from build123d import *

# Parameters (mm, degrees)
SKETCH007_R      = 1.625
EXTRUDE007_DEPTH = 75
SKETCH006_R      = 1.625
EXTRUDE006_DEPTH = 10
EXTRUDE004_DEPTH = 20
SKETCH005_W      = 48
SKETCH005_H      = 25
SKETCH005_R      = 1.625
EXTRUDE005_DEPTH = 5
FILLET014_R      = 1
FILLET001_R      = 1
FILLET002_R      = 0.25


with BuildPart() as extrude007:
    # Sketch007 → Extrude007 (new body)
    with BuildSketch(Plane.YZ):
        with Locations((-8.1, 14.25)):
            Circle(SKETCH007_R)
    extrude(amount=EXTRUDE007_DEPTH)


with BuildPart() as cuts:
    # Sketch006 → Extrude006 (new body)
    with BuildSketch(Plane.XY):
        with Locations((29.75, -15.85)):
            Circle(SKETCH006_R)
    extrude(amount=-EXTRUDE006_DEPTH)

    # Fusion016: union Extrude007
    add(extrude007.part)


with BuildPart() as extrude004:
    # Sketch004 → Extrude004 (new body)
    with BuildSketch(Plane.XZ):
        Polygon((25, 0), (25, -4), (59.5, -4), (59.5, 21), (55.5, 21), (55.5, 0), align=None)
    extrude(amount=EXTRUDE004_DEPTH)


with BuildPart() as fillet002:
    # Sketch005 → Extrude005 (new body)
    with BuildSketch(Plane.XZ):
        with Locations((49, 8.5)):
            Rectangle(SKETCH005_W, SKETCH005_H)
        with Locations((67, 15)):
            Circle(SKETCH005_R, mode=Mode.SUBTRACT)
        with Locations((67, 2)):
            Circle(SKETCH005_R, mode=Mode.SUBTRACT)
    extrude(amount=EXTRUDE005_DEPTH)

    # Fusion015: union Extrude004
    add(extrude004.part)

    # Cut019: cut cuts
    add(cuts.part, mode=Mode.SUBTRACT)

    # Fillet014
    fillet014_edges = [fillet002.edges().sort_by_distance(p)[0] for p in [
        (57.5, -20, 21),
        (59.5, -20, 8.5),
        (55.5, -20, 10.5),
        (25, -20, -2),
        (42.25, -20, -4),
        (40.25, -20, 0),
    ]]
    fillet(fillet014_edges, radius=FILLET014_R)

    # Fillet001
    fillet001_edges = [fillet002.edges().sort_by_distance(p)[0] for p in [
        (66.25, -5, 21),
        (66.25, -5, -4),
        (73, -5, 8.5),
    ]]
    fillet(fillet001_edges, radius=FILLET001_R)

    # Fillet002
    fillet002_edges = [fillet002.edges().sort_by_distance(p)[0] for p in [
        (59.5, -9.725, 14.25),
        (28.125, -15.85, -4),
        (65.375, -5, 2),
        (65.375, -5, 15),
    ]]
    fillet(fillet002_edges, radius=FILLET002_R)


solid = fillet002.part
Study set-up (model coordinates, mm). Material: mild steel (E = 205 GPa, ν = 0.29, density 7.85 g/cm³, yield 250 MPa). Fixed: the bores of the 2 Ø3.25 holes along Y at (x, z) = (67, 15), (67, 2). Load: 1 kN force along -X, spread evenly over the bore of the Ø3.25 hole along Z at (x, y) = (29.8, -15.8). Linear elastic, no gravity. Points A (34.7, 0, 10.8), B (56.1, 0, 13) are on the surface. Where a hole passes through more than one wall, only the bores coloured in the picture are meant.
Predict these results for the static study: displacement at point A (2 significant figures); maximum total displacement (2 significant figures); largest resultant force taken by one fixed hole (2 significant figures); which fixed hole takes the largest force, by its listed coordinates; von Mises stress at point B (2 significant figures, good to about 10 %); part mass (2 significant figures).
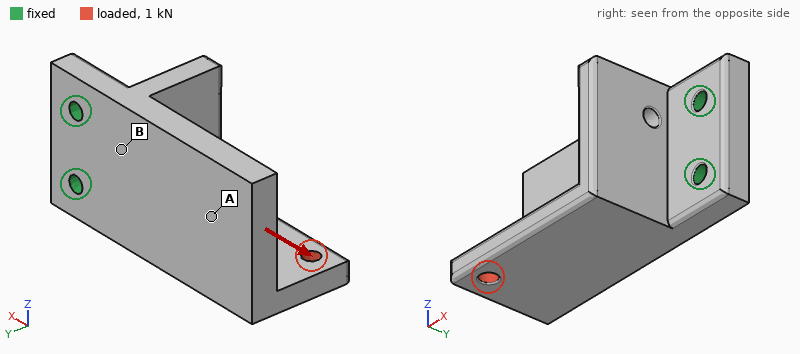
0.077 mm
0.13 mm
1.2 kN
(67, 2)
67 MPa
72 g
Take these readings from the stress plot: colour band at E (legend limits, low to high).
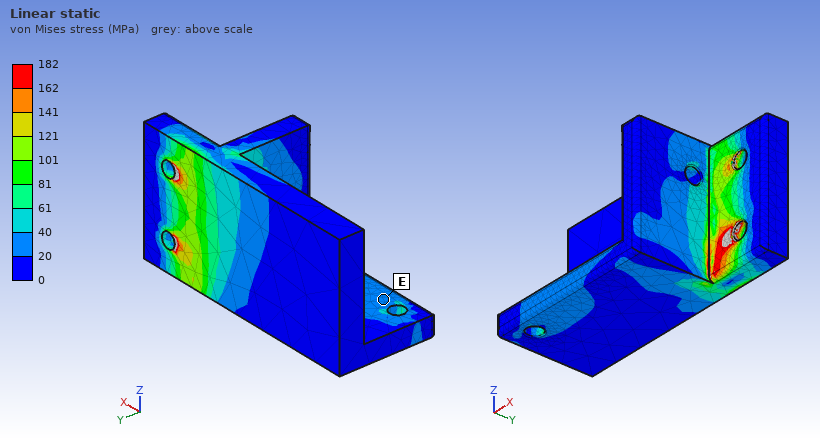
20 to 40 MPa
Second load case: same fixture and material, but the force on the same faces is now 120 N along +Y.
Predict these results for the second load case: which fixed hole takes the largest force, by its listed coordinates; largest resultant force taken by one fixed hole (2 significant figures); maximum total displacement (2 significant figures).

(67, 2)
130 N
39 µm
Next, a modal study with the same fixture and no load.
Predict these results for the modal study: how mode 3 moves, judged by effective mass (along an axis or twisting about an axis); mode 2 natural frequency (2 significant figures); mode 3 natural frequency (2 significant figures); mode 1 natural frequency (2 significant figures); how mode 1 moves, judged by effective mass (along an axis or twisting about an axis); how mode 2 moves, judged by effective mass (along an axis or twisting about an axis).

along Z
5800 Hz
7600 Hz
2100 Hz
along Y
along Z
